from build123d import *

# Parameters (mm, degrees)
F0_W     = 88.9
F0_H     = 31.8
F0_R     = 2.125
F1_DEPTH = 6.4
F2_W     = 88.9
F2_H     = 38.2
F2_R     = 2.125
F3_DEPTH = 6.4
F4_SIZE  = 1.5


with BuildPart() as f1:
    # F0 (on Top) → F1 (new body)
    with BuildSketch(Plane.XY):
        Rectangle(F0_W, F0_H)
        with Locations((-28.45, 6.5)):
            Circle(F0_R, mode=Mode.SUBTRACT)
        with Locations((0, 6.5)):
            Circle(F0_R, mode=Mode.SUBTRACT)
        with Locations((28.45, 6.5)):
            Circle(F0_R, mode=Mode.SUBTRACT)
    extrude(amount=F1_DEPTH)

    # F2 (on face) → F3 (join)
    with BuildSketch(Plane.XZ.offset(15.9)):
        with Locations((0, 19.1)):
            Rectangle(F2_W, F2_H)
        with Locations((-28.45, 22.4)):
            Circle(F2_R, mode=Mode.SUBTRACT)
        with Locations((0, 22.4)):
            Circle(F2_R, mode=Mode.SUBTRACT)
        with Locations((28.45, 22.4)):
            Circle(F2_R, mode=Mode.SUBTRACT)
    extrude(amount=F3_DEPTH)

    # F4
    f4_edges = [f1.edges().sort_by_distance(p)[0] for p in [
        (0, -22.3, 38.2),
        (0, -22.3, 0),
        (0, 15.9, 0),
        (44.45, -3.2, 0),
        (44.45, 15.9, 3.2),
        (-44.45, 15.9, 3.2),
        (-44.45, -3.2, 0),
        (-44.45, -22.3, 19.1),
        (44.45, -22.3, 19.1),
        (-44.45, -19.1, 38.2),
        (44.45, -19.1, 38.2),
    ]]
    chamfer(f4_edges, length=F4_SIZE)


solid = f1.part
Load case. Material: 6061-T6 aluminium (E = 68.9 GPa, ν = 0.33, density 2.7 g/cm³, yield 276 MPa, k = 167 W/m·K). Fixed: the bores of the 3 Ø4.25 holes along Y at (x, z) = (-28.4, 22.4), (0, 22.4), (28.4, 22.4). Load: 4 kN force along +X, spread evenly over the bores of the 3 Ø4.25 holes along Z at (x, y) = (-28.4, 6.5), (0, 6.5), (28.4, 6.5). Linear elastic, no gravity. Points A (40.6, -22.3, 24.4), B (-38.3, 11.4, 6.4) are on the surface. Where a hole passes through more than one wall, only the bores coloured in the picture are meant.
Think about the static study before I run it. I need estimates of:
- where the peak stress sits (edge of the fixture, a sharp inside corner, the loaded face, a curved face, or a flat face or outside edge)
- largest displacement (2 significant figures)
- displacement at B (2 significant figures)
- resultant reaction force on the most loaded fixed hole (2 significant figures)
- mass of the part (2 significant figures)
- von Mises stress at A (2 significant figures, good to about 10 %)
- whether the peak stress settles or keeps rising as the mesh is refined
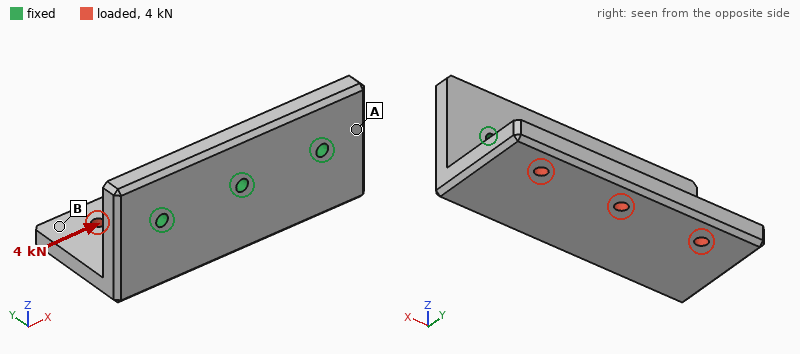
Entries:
edge of the fixture
0.16 mm
0.14 mm
2.4 kN
100 g
43 MPa
keeps rising
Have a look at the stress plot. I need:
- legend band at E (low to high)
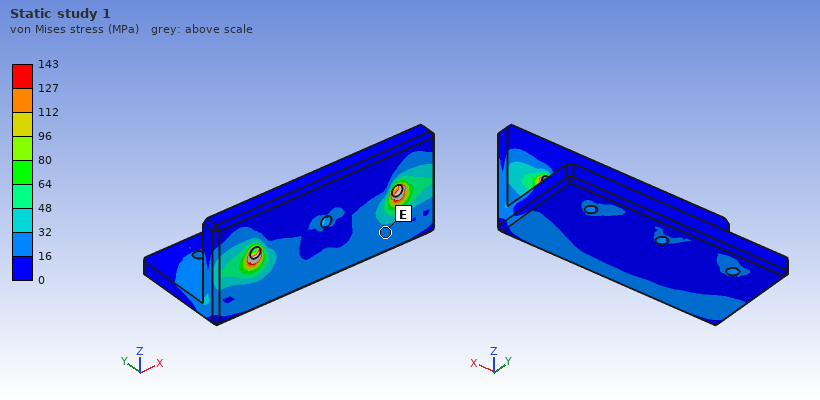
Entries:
16 to 32 MPa
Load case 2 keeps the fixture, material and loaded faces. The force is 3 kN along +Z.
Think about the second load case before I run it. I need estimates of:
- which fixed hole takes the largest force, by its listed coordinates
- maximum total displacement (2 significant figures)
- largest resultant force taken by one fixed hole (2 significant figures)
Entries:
(0, 22.4)
0.58 mm
1.2 kN
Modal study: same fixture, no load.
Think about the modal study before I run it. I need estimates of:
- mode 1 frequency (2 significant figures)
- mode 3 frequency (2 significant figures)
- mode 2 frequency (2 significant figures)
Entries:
2200 Hz
6000 Hz
3500 Hz
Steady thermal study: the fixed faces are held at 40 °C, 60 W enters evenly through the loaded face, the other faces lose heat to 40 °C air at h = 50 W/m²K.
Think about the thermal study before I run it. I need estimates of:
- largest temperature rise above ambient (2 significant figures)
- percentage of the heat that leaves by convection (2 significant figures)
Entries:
30 K
15 %
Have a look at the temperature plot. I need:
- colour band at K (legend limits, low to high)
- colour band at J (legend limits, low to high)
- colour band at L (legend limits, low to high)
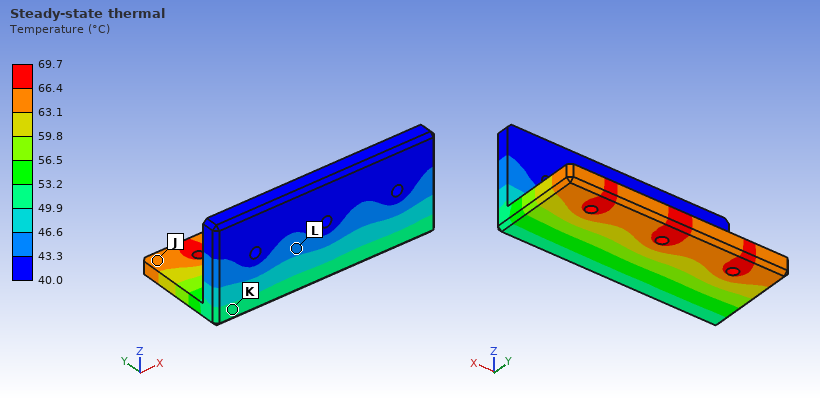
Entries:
49.9 to 53.2 °C
63.1 to 66.4 °C
43.3 to 46.6 °C
